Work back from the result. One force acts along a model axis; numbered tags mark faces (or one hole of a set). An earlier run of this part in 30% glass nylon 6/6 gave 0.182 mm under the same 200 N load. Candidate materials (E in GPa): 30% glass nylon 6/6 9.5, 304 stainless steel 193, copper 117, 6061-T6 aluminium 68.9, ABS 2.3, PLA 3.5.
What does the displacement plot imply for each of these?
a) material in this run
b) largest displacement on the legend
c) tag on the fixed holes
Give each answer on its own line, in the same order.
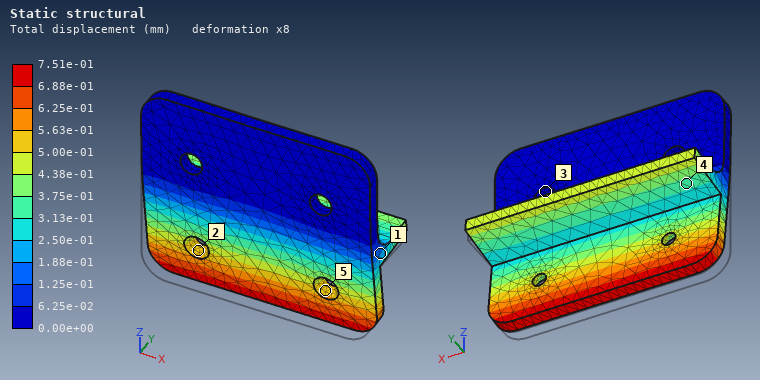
ABS
7.51e-01 mm
3
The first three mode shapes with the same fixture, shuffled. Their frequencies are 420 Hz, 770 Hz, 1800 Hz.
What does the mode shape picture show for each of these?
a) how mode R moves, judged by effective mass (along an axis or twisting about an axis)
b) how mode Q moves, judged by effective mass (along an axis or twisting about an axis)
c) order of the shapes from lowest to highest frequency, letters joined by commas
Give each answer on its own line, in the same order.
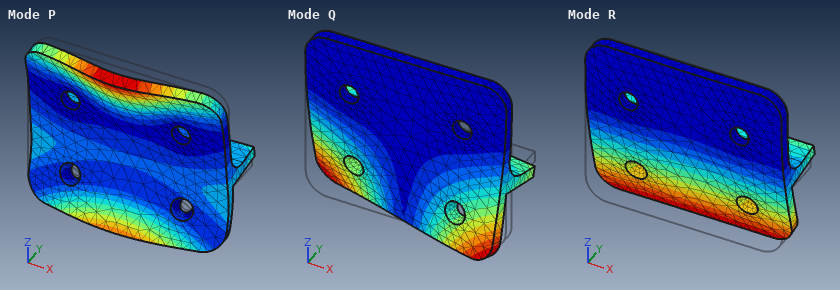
along Y
twisting about Z
R, Q, P
